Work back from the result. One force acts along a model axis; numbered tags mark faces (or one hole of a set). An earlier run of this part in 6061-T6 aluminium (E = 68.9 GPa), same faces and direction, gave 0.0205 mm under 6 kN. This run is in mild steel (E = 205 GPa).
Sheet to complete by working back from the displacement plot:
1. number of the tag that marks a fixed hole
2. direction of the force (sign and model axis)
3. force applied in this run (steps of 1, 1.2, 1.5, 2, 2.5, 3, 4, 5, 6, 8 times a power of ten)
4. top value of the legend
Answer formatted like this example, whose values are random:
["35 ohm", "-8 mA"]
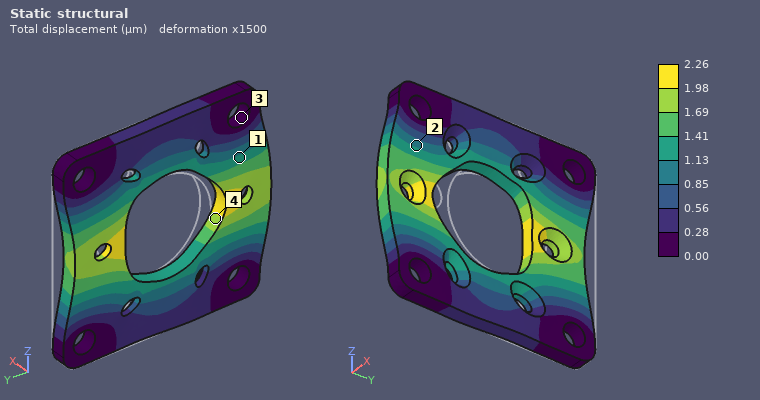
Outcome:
["3", "-Y", "2 kN", "2.26 µm"]
